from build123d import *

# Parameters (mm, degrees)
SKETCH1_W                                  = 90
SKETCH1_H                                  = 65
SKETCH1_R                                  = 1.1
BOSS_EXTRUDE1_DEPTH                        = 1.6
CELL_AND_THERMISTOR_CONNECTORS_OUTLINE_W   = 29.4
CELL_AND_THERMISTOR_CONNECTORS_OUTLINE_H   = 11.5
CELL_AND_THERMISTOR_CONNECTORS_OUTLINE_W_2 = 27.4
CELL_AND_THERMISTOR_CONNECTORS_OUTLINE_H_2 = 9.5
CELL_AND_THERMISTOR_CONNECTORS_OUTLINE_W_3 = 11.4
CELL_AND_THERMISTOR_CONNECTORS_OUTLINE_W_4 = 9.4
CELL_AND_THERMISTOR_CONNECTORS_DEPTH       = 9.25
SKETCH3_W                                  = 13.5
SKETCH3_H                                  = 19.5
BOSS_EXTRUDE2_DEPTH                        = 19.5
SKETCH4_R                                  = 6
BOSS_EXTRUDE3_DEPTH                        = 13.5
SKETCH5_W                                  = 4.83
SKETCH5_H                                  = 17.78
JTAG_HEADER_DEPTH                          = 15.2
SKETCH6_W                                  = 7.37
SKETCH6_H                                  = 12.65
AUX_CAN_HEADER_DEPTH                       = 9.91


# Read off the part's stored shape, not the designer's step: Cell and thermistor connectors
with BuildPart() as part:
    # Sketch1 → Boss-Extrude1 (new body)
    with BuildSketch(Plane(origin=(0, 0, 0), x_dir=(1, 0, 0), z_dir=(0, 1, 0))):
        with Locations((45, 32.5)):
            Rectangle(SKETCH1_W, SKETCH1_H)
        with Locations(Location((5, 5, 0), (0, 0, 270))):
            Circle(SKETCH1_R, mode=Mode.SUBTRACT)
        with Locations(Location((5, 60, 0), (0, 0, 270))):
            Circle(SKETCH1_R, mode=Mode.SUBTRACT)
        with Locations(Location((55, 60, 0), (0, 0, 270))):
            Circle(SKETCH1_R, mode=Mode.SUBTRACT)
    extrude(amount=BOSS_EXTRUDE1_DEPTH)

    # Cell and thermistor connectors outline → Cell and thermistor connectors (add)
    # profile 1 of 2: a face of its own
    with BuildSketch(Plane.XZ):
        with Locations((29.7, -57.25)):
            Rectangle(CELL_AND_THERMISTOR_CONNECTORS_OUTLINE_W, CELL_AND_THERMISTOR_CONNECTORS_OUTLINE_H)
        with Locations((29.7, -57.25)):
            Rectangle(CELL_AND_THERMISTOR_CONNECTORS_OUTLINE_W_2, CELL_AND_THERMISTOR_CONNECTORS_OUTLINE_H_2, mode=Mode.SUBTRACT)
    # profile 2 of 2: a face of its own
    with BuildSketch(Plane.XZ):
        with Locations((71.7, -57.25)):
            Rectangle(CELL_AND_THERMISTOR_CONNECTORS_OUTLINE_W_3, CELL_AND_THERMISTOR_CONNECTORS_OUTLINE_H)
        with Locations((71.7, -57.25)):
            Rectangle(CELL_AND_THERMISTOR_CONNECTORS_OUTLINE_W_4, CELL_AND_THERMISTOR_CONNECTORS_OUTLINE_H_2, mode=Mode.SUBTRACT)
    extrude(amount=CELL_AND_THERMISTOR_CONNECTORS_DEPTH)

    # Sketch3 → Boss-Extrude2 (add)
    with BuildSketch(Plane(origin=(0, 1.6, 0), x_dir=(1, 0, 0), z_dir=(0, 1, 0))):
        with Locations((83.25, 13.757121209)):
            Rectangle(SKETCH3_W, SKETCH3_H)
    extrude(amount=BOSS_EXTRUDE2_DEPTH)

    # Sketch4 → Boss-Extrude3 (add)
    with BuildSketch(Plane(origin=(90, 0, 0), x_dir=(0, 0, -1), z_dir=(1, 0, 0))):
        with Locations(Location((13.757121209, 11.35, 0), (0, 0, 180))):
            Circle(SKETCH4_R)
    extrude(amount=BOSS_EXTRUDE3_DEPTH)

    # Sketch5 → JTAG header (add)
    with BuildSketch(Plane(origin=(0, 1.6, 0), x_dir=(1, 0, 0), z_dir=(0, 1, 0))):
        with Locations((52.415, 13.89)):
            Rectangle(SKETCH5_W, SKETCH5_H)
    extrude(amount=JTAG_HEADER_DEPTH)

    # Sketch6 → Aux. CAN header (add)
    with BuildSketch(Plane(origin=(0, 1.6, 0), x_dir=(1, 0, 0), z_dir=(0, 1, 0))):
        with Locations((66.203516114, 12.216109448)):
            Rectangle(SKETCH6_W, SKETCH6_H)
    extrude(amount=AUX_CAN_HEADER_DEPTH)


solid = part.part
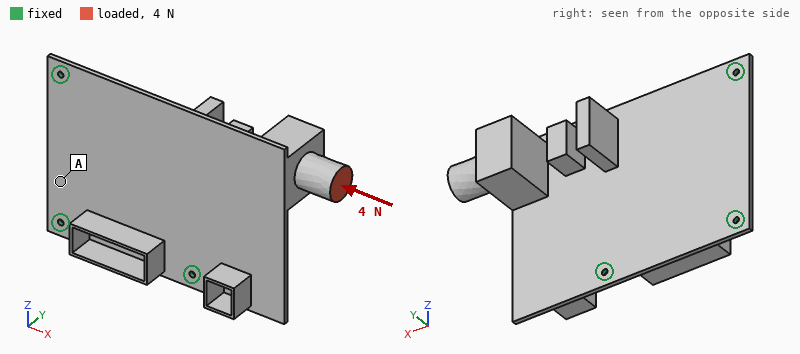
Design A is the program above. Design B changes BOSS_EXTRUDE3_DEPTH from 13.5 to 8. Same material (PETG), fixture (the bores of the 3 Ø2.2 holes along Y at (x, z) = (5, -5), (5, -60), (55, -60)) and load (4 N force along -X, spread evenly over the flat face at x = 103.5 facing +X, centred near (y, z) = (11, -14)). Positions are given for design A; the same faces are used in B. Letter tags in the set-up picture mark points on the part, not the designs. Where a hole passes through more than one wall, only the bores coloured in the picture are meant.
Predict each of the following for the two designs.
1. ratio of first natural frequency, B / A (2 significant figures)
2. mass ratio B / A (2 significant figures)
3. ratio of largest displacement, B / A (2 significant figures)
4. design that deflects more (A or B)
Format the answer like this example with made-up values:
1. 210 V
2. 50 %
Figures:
1. 1.1
2. 0.97
3. 0.90
4. A
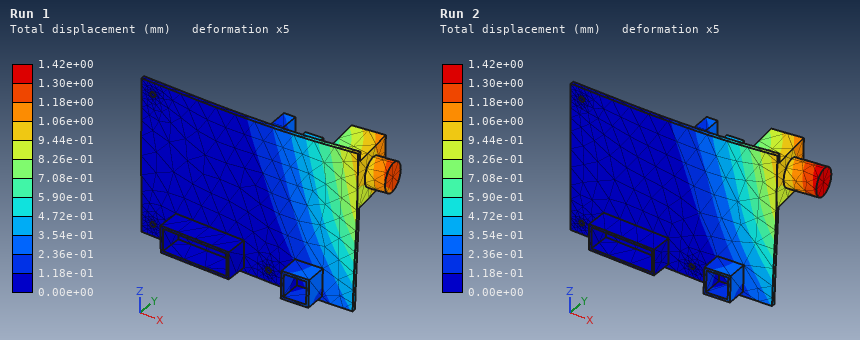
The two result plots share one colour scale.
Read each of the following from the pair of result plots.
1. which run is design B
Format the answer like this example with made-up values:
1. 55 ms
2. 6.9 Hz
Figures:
1. Run 1
